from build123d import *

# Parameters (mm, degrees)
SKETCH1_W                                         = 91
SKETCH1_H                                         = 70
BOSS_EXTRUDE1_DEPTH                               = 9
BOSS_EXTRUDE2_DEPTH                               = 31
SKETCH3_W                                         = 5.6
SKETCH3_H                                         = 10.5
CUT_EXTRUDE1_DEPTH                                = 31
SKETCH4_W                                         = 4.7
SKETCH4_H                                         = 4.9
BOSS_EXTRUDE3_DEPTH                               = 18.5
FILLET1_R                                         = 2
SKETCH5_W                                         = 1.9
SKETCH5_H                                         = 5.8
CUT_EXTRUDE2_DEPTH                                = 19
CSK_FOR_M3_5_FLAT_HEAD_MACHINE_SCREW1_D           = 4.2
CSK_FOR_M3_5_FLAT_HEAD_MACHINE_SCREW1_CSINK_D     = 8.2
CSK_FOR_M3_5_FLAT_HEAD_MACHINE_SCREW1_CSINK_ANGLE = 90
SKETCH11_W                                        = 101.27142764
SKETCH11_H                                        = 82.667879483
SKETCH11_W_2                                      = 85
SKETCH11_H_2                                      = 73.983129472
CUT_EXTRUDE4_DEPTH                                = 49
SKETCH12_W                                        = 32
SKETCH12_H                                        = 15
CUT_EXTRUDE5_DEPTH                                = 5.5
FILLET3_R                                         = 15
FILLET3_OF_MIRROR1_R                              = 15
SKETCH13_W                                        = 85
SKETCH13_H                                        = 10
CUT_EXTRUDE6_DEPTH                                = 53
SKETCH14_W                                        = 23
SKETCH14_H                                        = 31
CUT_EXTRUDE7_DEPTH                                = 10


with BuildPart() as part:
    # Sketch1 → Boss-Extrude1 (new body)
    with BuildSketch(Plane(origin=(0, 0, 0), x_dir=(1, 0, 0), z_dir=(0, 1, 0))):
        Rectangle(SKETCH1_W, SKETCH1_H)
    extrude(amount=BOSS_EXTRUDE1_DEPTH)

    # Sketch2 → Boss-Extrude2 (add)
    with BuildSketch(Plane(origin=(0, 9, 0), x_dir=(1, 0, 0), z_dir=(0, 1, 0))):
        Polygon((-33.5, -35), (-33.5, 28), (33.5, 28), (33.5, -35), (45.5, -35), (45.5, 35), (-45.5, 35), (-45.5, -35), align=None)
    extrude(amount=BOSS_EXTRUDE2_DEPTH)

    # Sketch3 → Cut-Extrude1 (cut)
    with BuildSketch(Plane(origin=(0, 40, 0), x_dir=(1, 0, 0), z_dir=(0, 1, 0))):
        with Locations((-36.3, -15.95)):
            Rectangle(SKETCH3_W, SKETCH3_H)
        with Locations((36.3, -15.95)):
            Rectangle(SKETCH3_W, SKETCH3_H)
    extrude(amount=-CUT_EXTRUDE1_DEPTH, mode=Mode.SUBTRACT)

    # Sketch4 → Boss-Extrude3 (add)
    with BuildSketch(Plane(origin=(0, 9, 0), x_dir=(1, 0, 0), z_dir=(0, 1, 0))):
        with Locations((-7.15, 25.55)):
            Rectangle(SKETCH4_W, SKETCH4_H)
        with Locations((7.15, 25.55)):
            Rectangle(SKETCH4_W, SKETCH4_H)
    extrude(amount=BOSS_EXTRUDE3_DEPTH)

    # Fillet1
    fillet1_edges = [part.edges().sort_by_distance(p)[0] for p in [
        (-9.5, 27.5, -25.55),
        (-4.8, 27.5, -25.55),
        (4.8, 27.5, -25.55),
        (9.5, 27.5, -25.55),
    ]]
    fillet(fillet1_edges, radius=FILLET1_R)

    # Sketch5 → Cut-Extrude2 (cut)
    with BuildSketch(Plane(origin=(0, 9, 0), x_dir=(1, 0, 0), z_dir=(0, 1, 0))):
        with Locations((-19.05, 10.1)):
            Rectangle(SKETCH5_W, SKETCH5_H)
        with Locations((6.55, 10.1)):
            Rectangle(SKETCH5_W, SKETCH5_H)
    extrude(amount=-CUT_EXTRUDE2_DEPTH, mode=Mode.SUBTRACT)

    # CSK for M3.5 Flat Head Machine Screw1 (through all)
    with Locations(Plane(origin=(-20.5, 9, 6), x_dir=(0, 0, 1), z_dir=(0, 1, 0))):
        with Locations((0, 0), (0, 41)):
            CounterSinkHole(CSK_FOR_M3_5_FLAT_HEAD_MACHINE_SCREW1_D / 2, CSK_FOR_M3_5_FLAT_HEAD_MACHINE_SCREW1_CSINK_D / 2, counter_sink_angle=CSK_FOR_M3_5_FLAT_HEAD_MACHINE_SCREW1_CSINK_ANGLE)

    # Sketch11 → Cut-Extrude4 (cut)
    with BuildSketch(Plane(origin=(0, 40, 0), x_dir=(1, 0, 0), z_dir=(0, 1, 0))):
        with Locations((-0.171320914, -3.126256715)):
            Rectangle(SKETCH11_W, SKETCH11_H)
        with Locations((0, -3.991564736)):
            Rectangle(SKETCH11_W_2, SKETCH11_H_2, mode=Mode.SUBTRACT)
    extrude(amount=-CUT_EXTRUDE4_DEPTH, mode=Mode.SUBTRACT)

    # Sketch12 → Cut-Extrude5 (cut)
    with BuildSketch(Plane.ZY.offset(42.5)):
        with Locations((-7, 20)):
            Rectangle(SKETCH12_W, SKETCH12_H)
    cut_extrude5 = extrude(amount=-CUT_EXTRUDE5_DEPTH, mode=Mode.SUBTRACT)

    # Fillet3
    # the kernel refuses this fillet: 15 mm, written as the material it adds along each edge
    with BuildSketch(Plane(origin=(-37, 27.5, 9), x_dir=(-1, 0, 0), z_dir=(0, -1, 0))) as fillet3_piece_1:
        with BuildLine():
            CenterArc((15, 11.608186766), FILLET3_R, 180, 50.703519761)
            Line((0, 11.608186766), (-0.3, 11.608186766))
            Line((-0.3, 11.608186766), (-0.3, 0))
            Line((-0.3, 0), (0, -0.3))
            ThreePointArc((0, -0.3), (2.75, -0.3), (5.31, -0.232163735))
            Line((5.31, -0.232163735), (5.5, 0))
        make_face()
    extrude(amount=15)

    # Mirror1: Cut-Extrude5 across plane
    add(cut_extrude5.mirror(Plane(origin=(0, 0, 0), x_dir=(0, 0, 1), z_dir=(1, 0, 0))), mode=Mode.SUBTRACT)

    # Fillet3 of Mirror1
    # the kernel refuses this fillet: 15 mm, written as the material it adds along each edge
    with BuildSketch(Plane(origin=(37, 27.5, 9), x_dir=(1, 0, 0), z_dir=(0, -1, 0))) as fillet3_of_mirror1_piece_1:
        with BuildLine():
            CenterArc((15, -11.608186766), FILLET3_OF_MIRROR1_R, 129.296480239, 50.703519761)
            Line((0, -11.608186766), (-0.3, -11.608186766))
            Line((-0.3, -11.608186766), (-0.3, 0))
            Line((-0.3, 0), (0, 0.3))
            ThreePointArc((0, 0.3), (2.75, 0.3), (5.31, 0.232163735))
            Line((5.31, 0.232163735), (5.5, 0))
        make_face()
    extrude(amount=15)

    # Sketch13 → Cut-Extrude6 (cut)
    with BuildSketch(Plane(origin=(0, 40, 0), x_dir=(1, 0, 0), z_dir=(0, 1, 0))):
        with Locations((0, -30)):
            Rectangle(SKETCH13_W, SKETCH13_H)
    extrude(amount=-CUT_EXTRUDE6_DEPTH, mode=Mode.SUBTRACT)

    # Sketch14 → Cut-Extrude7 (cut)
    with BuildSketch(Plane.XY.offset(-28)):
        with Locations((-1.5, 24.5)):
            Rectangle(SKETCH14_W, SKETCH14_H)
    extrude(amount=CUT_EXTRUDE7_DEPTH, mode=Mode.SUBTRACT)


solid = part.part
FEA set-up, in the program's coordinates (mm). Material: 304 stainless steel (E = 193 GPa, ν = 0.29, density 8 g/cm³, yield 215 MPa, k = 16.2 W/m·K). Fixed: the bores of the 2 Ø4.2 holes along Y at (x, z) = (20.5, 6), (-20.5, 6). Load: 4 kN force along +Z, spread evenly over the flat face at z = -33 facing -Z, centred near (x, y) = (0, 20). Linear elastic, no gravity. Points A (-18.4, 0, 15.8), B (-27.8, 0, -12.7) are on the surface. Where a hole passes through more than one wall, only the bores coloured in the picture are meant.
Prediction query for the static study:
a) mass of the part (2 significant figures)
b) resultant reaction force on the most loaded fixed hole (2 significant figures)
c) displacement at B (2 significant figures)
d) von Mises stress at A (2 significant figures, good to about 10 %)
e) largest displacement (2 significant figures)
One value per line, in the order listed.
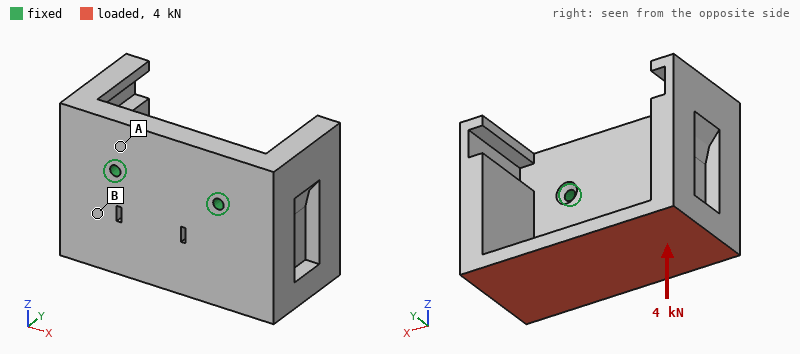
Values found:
630 g
2.0 kN
20 µm
27 MPa
95 µm
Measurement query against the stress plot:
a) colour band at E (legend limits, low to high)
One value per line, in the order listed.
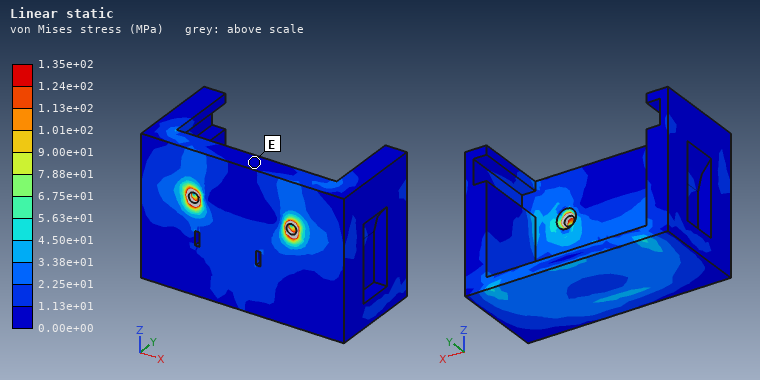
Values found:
0.00e+00 to 1.13e+01 MPa
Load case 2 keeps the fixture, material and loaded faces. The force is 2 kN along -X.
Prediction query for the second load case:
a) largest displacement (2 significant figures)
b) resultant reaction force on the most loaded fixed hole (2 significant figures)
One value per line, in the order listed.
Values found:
25 µm
2.2 kN
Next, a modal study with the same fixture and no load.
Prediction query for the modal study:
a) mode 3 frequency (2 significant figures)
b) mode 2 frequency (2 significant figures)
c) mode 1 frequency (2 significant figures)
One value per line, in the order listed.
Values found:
4100 Hz
2200 Hz
1700 Hz
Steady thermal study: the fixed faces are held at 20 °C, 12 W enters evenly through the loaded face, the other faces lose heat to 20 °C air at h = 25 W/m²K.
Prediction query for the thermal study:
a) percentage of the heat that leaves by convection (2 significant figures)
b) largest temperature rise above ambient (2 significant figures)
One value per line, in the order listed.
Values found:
56 %
32 K
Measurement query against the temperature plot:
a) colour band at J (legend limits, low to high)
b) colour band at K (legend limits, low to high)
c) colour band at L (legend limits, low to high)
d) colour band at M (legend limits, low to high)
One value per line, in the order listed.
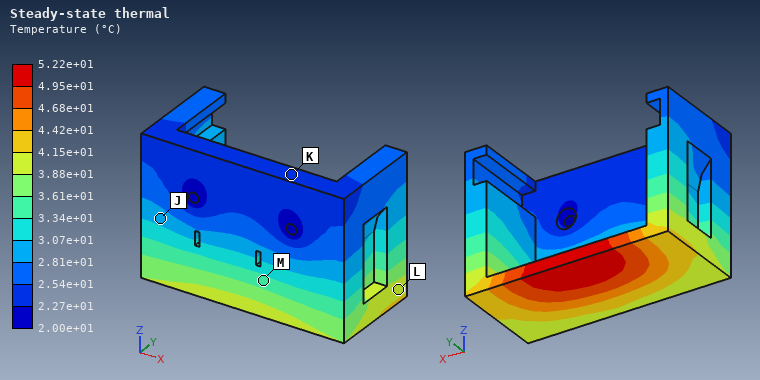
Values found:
2.81e+01 to 3.07e+01 °C
2.27e+01 to 2.54e+01 °C
3.88e+01 to 4.15e+01 °C
3.34e+01 to 3.61e+01 °C
